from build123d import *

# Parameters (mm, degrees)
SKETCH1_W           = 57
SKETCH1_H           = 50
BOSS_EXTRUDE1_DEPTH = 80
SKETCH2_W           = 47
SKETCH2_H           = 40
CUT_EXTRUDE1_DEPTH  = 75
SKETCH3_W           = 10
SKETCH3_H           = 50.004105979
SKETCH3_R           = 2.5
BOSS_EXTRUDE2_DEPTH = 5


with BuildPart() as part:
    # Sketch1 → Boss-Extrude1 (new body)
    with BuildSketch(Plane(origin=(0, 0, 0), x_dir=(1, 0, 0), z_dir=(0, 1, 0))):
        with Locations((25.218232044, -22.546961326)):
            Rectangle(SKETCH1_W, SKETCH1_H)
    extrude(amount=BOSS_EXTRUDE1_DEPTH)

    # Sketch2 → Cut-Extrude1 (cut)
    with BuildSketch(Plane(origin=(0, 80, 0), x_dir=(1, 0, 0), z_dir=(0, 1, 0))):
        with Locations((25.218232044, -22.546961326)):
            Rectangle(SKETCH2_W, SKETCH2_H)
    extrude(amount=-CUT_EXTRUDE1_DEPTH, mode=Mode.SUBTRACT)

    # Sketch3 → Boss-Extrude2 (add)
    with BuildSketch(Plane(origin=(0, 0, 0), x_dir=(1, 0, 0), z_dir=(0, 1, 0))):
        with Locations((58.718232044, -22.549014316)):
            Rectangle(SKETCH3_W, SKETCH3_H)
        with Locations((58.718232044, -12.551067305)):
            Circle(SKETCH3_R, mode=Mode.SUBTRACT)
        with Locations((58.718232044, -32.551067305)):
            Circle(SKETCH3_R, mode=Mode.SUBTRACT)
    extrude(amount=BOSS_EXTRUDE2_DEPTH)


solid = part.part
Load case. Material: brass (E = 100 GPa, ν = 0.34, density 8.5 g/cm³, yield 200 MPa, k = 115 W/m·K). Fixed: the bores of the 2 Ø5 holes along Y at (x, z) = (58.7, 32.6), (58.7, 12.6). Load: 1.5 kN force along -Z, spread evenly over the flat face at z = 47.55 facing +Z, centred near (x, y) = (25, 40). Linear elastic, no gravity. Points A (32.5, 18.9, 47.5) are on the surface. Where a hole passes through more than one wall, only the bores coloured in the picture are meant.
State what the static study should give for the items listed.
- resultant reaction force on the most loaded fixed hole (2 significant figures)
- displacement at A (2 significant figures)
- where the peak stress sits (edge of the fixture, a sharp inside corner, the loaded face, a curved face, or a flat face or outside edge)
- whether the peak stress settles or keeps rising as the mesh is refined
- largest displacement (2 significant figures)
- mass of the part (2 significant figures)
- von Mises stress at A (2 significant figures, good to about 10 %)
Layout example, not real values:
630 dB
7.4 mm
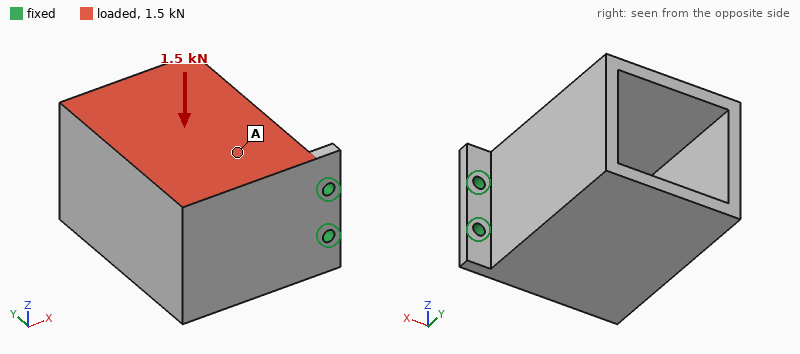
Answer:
3.1 kN
0.048 mm
edge of the fixture
keeps rising
0.15 mm
760 g
9.4 MPa
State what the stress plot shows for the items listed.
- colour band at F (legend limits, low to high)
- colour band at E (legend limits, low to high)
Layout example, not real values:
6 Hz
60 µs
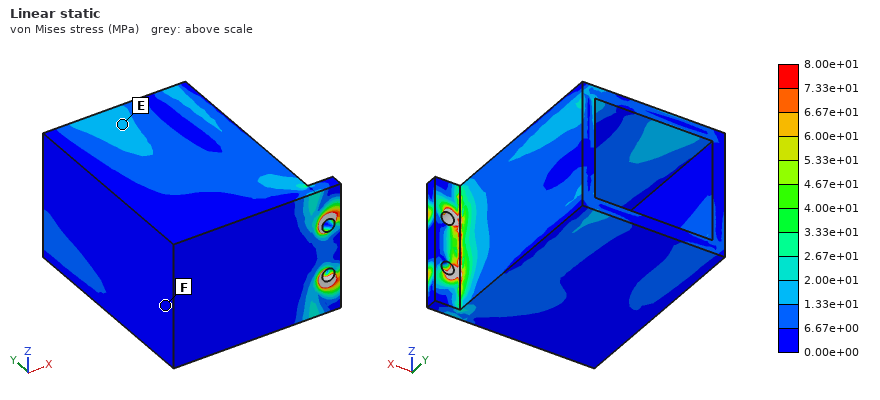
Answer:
0.00e+00 to 6.67e+00 MPa
1.33e+01 to 2.00e+01 MPa
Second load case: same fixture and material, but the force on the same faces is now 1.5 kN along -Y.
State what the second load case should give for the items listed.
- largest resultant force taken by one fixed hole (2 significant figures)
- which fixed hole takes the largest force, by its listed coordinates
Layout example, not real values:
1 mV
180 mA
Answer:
2.2 kN
(58.7, 32.6)
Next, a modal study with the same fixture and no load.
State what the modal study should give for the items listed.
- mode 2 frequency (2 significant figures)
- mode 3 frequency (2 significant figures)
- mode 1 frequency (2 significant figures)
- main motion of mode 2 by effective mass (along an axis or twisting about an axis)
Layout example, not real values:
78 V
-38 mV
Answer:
780 Hz
1700 Hz
250 Hz
along Z
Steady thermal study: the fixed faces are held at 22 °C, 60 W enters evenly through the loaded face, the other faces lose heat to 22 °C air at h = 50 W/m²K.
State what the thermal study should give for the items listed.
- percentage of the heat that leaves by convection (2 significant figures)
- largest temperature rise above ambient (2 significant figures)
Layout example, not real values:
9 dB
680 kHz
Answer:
53 %
37 K
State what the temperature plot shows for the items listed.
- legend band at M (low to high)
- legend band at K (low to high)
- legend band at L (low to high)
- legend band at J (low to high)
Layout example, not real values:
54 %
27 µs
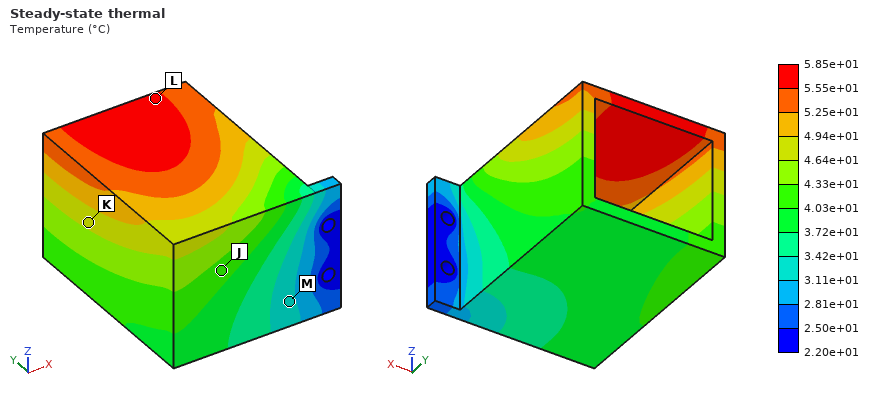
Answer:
3.11e+01 to 3.42e+01 °C
4.64e+01 to 4.94e+01 °C
5.55e+01 to 5.85e+01 °C
4.03e+01 to 4.33e+01 °C
